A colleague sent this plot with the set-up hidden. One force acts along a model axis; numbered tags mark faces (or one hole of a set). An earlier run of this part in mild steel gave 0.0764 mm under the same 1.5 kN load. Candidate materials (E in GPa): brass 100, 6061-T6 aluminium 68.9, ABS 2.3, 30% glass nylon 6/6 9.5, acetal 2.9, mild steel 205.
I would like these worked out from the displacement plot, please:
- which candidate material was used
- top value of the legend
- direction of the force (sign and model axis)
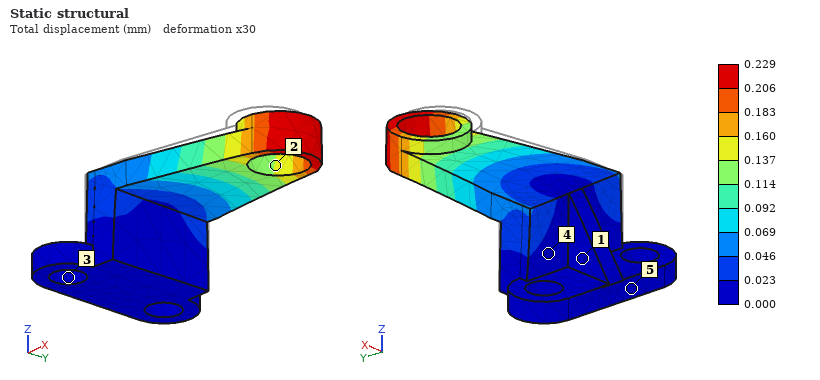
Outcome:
6061-T6 aluminium
0.229 mm
+Y
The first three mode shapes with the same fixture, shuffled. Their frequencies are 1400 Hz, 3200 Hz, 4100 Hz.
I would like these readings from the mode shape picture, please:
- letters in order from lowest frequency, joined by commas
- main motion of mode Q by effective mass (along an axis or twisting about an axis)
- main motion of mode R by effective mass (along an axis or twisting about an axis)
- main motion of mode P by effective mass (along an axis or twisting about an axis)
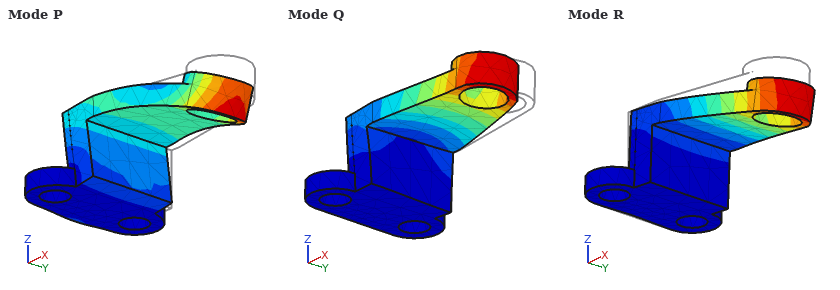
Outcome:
R, Q, P
along Y
along Z
along X
